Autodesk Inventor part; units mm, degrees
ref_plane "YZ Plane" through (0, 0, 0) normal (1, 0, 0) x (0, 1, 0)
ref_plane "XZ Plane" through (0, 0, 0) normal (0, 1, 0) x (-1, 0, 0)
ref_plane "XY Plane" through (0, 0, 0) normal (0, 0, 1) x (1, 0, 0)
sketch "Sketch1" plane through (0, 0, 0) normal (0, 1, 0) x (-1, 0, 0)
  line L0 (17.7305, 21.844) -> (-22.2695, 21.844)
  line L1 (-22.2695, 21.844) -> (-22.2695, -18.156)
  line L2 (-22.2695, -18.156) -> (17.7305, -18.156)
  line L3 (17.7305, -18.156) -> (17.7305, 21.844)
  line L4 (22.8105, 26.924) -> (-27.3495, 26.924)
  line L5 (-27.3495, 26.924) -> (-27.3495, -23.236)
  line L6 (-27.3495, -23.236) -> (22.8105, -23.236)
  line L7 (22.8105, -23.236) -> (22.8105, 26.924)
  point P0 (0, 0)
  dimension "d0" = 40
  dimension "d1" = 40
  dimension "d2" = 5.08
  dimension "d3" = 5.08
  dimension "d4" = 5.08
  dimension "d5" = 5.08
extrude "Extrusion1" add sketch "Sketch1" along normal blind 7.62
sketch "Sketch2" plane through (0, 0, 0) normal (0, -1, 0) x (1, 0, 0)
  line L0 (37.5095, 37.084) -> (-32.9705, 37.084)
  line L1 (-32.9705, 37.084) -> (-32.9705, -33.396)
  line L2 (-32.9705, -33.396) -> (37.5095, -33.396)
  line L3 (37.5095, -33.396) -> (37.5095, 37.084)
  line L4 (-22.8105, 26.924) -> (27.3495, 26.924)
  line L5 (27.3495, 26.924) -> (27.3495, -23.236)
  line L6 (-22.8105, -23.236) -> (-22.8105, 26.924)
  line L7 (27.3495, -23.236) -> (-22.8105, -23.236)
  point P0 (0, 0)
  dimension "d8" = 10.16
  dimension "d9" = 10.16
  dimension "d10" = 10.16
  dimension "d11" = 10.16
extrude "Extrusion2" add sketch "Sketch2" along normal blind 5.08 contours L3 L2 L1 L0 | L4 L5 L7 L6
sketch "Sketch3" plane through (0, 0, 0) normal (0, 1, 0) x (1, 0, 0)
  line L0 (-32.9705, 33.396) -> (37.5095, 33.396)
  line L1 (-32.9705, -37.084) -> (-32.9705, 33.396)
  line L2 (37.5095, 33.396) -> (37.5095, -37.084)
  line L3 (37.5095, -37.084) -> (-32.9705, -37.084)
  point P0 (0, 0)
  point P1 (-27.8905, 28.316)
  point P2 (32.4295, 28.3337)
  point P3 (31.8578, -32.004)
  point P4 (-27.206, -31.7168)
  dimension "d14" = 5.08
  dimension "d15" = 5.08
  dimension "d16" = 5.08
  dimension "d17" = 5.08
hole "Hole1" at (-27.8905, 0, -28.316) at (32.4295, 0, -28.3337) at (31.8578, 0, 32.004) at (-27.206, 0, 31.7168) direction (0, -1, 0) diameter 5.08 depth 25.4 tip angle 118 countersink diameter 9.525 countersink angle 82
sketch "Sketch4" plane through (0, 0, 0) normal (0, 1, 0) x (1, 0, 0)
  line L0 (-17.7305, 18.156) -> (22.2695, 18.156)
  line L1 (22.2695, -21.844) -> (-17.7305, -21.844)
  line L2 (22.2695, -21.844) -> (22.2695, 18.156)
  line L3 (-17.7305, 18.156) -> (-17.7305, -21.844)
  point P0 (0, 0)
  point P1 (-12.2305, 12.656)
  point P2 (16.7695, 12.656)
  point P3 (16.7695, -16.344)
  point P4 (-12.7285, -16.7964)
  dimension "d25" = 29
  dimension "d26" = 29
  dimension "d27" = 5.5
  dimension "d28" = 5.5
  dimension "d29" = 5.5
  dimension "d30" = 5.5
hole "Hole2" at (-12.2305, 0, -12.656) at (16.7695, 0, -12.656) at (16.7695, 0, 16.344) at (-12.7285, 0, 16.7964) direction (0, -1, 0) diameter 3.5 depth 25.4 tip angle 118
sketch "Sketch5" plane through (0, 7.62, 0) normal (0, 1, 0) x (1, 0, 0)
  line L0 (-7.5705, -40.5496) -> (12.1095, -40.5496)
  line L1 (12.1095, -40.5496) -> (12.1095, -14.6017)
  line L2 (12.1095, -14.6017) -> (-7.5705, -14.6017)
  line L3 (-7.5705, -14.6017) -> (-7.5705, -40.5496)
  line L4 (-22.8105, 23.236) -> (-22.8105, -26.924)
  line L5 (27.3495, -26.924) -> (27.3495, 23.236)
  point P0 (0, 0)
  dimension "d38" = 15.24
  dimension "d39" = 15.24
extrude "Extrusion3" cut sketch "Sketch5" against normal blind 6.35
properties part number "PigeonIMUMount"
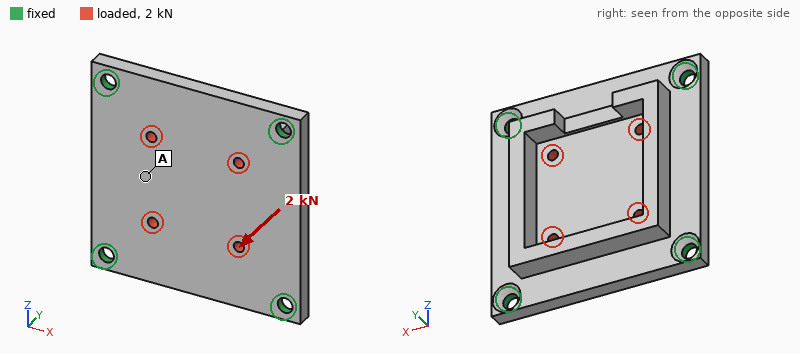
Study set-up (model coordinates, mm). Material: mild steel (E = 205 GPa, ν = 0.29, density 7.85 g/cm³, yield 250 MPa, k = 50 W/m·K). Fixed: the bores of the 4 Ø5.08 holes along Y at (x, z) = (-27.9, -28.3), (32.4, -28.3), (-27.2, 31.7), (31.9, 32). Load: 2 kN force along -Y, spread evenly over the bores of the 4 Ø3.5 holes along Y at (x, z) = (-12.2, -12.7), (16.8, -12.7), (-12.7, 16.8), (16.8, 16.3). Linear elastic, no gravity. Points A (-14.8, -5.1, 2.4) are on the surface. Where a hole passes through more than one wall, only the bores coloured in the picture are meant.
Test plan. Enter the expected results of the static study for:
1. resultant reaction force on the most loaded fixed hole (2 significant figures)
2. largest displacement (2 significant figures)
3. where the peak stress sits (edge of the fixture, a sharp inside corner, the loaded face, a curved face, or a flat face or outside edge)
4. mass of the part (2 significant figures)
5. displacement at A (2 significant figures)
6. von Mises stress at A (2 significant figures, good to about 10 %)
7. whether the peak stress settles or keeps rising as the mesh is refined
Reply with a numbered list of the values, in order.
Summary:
1. 820 N
2. 15 µm
3. edge of the fixture
4. 240 g
5. 11 µm
6. 10 MPa
7. keeps rising
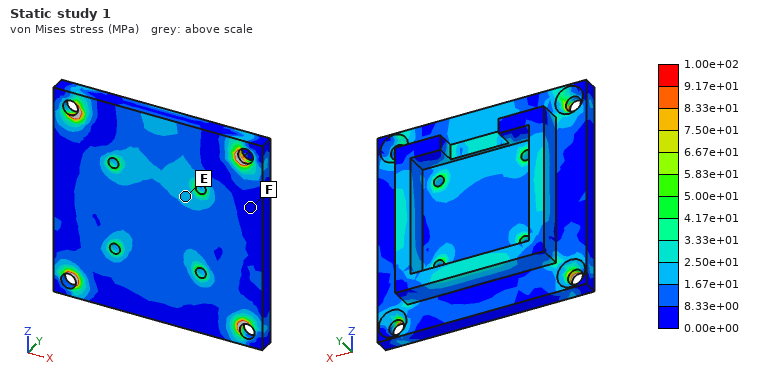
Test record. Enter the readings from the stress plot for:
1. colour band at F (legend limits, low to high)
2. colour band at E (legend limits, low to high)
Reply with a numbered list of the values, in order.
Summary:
1. 0.00e+00 to 8.33e+00 MPa
2. 1.67e+01 to 2.50e+01 MPa
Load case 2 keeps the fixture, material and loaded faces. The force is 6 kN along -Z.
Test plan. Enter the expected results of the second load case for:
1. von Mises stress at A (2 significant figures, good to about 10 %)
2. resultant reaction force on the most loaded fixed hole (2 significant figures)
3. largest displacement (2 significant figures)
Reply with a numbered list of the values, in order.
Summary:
1. 11 MPa
2. 1.6 kN
3. 3.7 µm
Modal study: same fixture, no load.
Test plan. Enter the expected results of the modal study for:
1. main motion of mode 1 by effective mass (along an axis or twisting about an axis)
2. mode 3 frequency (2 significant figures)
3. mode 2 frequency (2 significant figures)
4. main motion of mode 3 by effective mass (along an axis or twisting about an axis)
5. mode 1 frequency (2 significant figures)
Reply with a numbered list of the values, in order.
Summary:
1. along Y
2. 8800 Hz
3. 8000 Hz
4. twisting about Z
5. 5200 Hz
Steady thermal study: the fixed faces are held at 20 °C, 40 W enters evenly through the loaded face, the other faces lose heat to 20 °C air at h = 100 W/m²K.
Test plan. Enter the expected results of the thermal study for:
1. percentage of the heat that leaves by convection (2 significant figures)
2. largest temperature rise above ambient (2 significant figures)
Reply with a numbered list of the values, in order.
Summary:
1. 49 %
2. 29 K
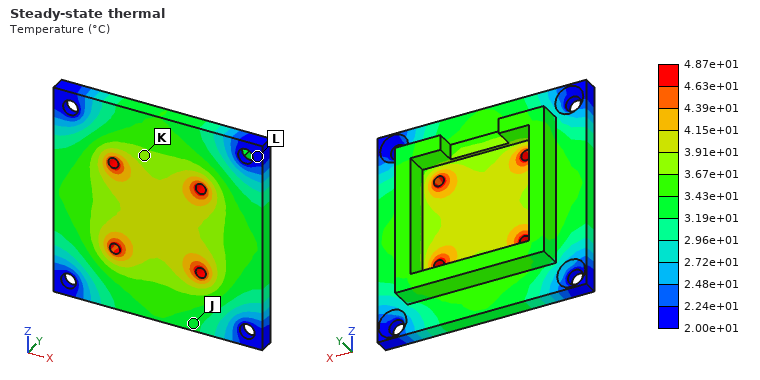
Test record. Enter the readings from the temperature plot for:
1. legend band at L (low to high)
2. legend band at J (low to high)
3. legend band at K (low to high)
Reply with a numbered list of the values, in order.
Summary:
1. 2.00e+01 to 2.24e+01 °C
2. 3.19e+01 to 3.43e+01 °C
3. 3.67e+01 to 3.91e+01 °C
